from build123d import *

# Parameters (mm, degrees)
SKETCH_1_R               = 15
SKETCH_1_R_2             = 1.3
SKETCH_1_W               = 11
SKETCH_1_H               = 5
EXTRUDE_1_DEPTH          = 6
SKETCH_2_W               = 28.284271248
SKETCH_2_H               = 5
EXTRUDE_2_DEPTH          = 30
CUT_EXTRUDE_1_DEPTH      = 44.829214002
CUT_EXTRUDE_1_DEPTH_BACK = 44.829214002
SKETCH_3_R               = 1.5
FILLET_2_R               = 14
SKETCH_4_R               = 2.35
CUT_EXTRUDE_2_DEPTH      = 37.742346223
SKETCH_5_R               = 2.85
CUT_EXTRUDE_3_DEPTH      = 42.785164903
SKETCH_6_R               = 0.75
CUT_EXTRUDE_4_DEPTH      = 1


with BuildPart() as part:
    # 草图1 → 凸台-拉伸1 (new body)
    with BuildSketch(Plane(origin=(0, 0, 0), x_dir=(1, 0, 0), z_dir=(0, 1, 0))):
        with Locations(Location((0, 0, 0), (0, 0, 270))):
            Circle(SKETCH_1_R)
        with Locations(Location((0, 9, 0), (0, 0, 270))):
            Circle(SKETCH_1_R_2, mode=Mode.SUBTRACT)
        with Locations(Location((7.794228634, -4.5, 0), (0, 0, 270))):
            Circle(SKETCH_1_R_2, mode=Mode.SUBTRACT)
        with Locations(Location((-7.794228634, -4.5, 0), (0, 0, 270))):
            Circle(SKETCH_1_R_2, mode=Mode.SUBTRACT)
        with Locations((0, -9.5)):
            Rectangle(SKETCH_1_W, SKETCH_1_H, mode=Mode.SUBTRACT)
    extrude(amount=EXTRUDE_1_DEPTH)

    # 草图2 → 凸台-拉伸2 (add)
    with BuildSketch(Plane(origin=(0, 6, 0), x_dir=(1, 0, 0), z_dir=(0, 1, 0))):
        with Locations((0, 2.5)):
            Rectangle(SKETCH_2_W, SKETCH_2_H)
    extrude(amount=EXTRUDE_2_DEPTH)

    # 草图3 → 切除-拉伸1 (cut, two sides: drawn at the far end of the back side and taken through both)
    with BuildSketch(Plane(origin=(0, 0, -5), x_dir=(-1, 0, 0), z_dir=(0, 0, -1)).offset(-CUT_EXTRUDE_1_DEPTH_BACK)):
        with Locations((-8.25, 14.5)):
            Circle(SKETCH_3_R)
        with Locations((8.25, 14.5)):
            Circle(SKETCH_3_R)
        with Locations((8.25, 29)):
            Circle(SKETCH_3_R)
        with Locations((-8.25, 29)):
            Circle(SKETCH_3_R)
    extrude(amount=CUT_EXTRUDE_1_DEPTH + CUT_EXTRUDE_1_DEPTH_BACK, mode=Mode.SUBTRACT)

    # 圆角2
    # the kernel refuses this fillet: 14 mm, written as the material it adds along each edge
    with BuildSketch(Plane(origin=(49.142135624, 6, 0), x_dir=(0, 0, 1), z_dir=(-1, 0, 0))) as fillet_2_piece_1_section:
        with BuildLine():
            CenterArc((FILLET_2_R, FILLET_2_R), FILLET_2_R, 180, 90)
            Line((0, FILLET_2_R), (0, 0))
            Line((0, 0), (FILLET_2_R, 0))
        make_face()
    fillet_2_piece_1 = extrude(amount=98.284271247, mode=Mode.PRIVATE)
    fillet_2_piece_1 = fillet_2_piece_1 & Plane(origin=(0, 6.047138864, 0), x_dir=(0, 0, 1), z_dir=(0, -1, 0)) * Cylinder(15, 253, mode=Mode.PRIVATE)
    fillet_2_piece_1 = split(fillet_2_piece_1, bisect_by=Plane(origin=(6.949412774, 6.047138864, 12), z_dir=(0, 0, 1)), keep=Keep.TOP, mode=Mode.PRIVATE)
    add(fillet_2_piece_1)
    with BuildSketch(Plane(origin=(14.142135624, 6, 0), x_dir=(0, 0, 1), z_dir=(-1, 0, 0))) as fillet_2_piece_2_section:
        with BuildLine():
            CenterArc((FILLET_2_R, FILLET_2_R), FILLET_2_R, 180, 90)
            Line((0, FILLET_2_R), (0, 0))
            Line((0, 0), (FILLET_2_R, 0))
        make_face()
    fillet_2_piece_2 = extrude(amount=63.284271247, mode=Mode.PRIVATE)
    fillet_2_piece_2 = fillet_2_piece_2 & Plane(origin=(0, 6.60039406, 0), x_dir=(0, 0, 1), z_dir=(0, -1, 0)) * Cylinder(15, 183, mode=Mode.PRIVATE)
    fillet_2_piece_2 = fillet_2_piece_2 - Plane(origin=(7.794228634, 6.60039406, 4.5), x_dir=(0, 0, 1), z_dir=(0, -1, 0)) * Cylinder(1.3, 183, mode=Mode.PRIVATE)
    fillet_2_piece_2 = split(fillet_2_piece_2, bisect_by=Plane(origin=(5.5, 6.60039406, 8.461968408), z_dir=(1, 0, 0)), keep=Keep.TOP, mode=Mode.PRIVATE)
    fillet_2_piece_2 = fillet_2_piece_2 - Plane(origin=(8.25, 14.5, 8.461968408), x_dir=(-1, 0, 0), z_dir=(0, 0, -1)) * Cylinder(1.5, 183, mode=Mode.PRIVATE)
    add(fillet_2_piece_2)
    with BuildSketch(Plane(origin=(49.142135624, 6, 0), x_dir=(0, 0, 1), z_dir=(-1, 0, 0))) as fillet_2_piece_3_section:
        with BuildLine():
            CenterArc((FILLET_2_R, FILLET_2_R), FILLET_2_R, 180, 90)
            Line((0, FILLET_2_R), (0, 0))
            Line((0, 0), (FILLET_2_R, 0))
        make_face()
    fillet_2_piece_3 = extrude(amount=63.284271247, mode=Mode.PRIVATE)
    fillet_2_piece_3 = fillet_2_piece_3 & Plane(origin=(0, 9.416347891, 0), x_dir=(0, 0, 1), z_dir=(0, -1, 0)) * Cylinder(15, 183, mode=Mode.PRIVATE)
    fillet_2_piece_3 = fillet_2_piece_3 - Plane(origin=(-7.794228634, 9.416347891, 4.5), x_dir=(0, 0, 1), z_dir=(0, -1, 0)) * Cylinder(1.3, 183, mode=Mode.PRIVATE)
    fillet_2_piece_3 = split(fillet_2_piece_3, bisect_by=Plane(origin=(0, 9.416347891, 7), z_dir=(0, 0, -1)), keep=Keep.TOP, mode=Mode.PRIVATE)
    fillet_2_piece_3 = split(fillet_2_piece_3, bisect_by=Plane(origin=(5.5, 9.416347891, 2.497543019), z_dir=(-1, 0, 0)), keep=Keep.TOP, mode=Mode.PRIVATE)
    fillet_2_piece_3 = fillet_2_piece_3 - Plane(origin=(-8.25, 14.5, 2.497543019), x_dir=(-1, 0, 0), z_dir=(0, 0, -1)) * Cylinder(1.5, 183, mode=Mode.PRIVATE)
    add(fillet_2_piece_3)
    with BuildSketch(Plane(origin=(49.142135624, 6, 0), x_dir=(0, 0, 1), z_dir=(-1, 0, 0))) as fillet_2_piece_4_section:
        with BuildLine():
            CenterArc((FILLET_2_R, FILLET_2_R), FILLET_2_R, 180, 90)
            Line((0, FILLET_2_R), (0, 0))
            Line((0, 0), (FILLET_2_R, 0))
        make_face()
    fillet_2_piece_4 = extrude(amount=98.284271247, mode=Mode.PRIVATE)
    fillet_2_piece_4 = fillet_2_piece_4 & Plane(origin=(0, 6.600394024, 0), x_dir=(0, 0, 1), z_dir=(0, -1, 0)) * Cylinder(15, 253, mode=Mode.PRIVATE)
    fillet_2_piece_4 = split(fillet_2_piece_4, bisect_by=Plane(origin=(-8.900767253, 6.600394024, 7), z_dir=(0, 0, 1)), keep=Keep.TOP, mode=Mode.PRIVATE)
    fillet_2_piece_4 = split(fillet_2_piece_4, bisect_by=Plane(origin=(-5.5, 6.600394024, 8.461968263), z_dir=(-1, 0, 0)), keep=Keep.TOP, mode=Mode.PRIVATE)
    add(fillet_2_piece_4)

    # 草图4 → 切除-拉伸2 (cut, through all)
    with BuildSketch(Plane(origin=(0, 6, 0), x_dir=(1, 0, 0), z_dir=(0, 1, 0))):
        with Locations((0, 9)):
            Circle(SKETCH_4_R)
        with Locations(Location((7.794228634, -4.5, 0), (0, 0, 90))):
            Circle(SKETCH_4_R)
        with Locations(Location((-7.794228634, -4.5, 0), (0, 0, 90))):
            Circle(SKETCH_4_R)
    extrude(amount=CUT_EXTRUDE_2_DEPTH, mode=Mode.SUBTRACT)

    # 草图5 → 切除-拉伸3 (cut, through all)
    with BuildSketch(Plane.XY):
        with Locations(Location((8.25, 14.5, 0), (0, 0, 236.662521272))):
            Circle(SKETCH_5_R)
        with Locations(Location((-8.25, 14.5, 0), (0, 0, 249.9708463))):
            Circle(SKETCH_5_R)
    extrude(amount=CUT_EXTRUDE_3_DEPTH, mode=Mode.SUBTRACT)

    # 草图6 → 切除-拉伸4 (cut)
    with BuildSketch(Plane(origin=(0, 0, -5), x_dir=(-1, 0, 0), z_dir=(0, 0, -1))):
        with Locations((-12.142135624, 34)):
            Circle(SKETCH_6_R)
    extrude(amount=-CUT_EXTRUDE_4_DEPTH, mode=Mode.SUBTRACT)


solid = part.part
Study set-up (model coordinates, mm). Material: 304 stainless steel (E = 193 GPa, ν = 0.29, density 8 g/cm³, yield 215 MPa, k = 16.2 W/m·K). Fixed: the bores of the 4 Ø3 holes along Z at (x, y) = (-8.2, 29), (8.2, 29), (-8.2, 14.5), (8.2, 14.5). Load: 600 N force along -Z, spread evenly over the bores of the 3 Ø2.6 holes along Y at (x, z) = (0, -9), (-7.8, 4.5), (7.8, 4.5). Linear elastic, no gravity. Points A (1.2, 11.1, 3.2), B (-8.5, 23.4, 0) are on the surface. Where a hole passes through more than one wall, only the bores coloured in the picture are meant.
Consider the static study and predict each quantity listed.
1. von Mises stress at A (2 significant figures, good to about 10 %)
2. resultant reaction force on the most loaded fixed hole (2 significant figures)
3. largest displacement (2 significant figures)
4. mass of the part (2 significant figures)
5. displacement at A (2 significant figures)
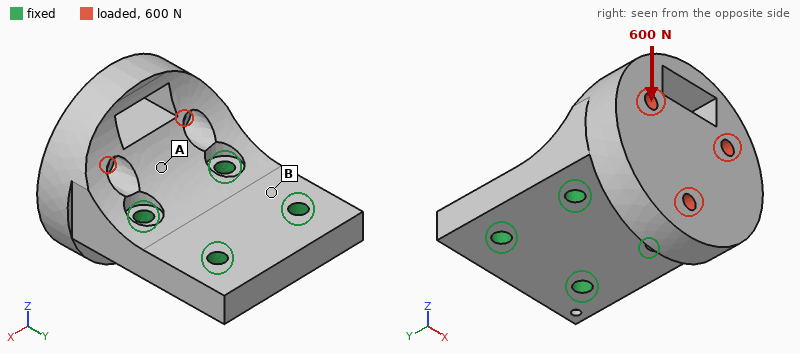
13 MPa
380 N
8.8 µm
71 g
2.2 µm
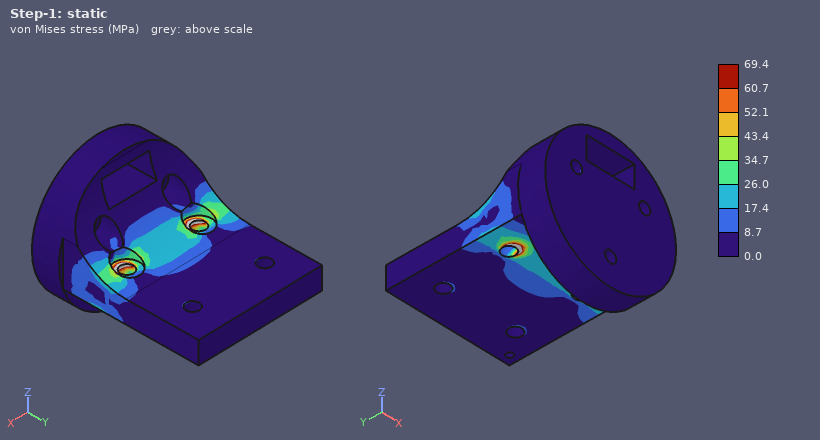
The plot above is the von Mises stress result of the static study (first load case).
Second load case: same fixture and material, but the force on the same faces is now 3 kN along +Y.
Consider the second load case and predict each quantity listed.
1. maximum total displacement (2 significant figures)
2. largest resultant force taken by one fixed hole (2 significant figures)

11 µm
1.3 kN
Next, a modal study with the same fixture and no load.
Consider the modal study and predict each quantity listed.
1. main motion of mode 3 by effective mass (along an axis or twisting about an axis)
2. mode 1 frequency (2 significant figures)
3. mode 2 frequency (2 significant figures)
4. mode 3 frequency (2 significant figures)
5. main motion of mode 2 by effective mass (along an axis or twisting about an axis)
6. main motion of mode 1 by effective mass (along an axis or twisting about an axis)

along X
8300 Hz
17 kHz
22 kHz
twisting about Y
along Z
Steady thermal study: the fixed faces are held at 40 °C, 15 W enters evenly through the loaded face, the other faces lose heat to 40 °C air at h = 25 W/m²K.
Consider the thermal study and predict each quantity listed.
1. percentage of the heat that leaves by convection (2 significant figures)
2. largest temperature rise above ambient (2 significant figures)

18 %
63 K
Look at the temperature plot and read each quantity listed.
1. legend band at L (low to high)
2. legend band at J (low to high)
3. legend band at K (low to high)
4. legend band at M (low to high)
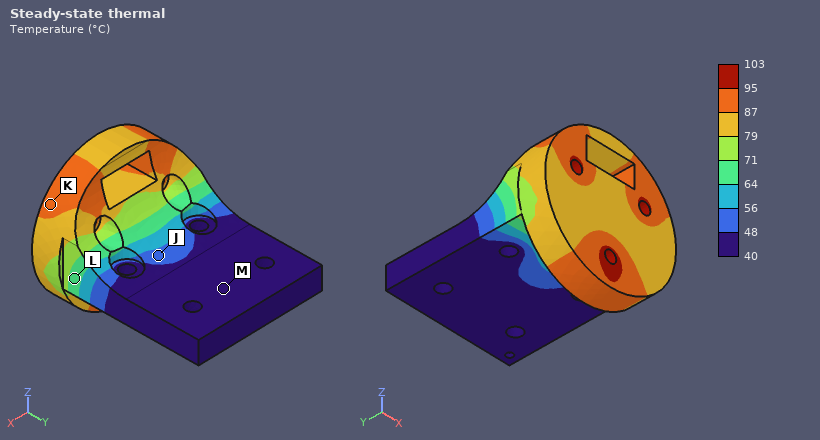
64 to 71 °C
48 to 56 °C
87 to 95 °C
40 to 48 °C
